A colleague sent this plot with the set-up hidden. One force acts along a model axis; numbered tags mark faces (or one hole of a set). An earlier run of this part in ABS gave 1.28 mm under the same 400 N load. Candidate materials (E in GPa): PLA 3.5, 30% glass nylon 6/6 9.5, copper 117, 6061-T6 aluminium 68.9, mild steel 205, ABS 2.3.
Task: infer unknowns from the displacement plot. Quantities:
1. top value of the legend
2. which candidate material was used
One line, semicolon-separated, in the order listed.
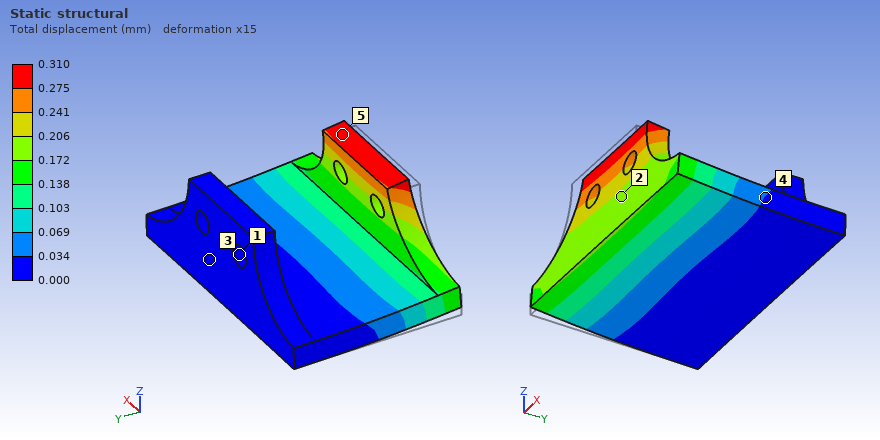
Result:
0.310 mm; 30% glass nylon 6/6
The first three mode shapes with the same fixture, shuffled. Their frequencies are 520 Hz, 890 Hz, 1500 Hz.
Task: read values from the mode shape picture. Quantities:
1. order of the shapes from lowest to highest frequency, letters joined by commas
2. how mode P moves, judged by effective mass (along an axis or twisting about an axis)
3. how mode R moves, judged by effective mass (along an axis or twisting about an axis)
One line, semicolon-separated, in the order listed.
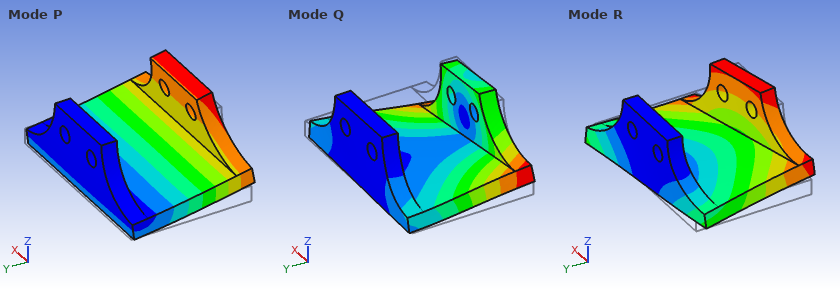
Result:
P, R, Q; along Z; along X
